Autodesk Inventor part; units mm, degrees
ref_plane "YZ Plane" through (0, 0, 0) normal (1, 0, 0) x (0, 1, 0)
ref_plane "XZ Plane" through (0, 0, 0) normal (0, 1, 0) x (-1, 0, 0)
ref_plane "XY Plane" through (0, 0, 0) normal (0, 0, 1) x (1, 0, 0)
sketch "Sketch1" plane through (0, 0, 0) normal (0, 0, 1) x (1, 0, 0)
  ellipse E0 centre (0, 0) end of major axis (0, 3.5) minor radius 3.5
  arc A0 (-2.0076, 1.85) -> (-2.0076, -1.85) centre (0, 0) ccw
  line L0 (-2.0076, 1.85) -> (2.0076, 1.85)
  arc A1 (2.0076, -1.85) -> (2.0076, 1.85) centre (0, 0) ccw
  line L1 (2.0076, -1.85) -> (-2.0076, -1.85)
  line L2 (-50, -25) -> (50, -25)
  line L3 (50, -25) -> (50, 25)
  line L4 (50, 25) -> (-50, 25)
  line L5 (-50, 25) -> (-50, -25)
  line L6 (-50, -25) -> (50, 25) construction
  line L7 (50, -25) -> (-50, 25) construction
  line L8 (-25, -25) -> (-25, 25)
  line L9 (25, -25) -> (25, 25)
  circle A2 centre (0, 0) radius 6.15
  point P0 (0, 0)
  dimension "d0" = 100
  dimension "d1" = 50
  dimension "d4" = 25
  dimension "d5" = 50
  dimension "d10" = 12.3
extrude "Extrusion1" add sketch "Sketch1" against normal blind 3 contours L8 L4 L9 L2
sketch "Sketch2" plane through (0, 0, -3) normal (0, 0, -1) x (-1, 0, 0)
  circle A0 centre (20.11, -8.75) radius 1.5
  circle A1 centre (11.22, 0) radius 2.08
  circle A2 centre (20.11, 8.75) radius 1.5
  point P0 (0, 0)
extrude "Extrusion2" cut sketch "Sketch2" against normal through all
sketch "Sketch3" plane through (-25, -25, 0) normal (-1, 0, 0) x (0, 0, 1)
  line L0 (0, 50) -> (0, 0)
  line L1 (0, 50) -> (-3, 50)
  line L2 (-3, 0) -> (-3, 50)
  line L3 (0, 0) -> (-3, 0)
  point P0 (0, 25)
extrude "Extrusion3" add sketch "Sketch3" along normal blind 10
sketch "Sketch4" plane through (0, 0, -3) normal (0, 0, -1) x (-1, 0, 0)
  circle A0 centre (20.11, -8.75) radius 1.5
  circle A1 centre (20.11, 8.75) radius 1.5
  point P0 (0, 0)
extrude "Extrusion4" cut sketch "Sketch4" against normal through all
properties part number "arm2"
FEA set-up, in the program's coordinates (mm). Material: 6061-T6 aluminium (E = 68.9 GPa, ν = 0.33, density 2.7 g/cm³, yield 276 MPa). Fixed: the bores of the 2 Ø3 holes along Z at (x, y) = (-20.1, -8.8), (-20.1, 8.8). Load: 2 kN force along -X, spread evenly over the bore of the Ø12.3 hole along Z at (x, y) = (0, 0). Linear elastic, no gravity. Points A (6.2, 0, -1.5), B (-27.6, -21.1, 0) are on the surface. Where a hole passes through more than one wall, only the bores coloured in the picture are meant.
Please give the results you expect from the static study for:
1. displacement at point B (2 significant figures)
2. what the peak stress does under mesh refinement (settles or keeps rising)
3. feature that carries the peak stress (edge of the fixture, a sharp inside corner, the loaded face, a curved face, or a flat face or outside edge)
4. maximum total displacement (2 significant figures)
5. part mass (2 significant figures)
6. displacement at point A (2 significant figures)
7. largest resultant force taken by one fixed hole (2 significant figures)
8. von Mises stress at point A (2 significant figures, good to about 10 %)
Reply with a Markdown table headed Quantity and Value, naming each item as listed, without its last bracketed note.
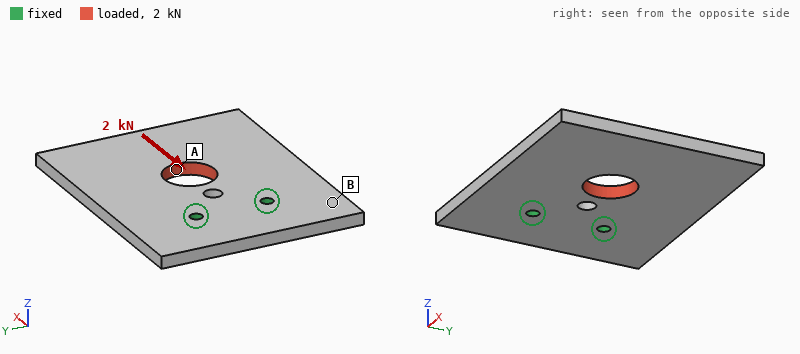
| Quantity | Value |
|---|---|
| displacement at point B | 3.6 µm |
| what the peak stress does under mesh refinement | keeps rising |
| feature that carries the peak stress | edge of the fixture |
| maximum total displacement | 11 µm |
| part mass | 23 g |
| displacement at point A | 11 µm |
| largest resultant force taken by one fixed hole | 1.0 kN |
| von Mises stress at point A | 19 MPa |
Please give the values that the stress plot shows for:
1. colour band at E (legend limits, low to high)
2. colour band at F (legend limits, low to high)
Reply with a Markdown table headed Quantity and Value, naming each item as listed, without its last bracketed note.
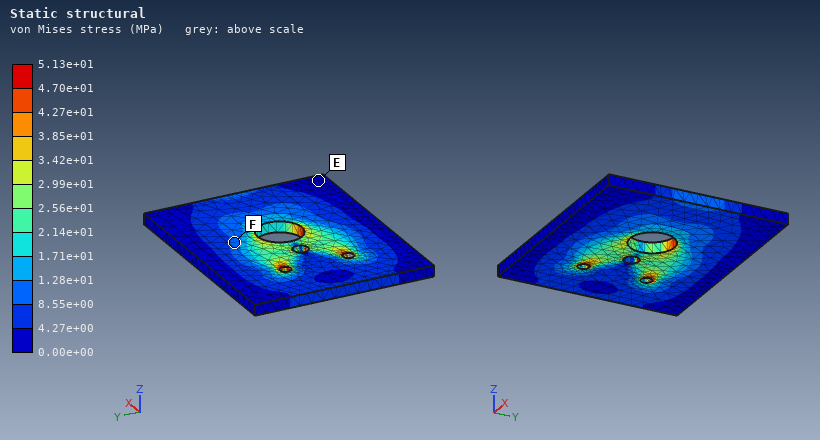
| Quantity | Value |
|---|---|
| colour band at E | 0.00e+00 to 4.27e+00 MPa |
| colour band at F | 8.55e+00 to 1.28e+01 MPa |
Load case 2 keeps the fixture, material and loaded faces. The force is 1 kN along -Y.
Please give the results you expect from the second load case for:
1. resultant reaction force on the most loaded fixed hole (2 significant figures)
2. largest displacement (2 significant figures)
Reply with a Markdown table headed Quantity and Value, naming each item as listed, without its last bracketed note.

| Quantity | Value |
|---|---|
| resultant reaction force on the most loaded fixed hole | 1.1 kN |
| largest displacement | 36 µm |
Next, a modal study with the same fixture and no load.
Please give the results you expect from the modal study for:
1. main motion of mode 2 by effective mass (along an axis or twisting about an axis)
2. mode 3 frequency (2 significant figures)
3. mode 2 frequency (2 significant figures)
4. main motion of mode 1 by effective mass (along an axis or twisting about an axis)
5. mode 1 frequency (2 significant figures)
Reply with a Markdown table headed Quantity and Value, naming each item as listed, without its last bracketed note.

| Quantity | Value |
|---|---|
| main motion of mode 2 by effective mass | twisting about X |
| mode 3 frequency | 5800 Hz |
| mode 2 frequency | 2300 Hz |
| main motion of mode 1 by effective mass | along Z |
| mode 1 frequency | 1100 Hz |
